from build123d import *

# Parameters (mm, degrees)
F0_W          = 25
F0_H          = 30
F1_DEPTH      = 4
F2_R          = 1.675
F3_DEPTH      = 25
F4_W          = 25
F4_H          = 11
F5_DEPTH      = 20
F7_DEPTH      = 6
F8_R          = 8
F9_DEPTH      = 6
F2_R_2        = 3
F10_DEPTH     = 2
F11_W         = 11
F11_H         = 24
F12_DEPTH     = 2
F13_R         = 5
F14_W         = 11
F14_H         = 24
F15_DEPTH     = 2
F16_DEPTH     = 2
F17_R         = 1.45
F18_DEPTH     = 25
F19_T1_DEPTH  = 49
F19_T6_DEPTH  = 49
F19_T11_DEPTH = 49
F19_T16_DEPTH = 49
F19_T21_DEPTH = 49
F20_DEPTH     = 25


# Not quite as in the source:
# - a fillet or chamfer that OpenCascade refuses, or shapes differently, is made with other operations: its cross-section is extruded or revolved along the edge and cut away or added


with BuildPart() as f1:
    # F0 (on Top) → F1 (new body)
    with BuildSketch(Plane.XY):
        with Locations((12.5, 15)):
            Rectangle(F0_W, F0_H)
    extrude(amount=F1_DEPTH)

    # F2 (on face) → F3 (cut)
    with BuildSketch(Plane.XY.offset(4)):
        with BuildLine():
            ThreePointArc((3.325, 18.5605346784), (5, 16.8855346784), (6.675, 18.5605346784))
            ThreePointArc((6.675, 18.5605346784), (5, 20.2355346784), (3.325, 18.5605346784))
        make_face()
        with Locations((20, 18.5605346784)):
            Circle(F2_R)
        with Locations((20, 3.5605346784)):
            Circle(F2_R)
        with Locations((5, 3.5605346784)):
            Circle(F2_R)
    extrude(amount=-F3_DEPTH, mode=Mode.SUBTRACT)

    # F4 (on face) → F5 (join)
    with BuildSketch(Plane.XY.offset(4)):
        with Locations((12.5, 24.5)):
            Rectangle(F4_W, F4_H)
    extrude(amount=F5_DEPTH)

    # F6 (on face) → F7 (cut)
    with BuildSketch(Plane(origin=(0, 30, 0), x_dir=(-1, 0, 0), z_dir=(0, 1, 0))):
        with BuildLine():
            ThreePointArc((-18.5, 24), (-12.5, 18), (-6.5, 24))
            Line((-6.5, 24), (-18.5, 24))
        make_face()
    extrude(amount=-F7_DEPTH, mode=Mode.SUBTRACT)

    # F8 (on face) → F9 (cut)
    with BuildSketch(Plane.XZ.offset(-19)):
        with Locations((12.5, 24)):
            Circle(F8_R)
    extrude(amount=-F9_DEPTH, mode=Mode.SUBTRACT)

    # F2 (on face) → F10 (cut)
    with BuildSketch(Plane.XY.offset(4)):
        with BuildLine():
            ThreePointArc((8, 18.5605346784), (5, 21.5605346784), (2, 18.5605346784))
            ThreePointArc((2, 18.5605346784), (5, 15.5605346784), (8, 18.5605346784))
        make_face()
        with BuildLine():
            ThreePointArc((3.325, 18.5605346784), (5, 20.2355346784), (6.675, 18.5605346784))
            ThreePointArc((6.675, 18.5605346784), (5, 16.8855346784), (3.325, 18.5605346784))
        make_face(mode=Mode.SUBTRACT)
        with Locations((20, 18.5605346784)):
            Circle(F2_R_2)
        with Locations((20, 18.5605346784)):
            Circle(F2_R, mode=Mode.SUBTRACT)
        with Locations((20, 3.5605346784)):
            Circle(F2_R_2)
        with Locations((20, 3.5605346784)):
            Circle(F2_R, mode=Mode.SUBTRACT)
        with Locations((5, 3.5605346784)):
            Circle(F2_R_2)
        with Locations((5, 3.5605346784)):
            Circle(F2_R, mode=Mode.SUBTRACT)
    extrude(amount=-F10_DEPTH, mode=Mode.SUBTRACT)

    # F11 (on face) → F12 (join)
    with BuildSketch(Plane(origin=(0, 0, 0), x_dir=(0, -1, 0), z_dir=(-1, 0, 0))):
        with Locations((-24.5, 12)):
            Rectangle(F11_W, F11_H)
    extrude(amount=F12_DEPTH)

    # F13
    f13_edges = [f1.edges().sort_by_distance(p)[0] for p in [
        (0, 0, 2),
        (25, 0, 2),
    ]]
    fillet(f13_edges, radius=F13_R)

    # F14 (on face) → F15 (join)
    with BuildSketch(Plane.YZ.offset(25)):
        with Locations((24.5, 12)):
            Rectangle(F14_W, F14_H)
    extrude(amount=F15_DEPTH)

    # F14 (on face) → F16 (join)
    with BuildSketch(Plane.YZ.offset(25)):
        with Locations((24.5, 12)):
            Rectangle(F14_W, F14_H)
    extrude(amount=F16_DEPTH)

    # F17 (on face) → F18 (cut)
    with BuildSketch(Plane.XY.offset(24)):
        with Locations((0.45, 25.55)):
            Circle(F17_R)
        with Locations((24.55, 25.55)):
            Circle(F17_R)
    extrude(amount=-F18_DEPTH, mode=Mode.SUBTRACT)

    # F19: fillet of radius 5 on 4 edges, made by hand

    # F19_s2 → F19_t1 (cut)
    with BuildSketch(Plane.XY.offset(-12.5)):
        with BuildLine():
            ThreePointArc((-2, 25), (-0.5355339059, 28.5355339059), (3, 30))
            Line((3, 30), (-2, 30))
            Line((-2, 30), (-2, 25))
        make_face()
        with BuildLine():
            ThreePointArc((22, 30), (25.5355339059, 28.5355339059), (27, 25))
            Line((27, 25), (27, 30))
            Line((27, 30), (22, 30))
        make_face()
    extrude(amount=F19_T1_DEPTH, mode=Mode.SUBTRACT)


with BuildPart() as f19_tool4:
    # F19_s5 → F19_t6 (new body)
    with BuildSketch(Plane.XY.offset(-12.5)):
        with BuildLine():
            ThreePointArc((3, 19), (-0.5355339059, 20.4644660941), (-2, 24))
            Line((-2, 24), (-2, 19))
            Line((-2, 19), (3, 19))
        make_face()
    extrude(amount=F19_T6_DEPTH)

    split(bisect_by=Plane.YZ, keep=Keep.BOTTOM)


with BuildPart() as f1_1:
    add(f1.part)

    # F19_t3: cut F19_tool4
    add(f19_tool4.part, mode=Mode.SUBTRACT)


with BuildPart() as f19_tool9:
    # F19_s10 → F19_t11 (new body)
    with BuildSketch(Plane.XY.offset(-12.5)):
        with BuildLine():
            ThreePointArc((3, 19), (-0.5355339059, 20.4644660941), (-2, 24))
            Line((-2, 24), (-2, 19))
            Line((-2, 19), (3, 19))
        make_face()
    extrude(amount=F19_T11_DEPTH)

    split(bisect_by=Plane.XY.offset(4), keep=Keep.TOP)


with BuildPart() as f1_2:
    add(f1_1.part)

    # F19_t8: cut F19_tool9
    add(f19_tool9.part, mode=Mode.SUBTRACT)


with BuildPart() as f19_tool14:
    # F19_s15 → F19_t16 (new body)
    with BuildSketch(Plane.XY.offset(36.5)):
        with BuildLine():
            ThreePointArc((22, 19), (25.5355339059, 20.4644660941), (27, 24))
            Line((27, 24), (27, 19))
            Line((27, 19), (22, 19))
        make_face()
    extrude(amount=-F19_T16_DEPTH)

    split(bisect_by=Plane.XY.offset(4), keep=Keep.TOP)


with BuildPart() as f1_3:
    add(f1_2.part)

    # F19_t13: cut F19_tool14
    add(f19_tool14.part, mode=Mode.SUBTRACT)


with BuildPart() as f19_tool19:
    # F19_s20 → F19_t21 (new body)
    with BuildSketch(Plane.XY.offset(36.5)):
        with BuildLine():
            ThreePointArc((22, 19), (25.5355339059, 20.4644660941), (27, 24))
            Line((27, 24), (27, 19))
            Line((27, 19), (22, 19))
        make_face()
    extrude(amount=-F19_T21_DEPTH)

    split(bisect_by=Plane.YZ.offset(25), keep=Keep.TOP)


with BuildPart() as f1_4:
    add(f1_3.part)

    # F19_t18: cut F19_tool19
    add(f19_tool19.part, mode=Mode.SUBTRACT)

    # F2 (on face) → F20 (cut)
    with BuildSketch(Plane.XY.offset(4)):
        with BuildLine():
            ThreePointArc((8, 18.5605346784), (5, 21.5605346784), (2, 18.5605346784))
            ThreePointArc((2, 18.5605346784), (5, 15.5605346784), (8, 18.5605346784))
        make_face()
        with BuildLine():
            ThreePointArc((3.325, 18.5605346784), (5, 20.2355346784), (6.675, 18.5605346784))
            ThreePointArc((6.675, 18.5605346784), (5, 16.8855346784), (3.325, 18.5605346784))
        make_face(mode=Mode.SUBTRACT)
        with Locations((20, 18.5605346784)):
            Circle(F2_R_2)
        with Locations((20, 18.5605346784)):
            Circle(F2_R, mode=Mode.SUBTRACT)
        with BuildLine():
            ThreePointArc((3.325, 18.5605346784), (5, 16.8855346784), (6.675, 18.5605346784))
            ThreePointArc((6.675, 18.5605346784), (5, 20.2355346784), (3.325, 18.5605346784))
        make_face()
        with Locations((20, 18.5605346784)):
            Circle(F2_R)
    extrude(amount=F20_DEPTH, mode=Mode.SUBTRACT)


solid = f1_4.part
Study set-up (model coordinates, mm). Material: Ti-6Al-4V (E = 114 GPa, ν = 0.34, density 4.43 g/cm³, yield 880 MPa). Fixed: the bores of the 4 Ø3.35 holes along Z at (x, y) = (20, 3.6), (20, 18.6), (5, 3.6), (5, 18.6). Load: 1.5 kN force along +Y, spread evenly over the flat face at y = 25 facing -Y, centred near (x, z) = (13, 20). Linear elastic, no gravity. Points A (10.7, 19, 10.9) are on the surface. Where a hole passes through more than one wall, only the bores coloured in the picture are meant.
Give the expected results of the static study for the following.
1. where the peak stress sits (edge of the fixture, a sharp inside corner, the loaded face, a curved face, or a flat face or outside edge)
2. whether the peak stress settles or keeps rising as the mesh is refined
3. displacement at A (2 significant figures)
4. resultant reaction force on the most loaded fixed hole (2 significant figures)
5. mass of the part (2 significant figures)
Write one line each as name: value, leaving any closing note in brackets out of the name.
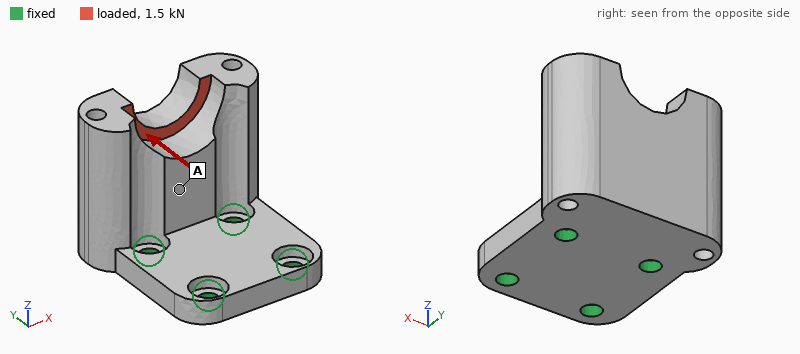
where the peak stress sits: edge of the fixture
whether the peak stress settles or keeps rising as the mesh is refined: keeps rising
displacement at A: 0.089 mm
resultant reaction force on the most loaded fixed hole: 1.3 kN
mass of the part: 31 g
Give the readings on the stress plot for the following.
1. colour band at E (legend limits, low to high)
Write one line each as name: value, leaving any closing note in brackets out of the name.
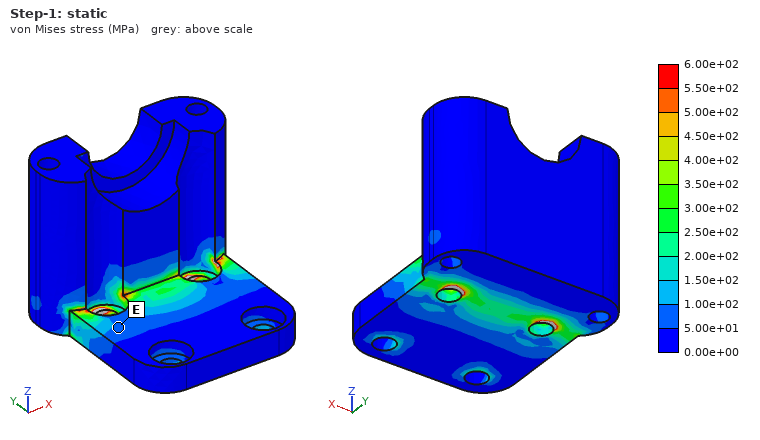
colour band at E: 5.00e+01 to 1.00e+02 MPa
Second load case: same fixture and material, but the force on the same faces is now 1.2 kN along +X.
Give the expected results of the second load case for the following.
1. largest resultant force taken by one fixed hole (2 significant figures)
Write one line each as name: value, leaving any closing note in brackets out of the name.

largest resultant force taken by one fixed hole: 1.5 kN
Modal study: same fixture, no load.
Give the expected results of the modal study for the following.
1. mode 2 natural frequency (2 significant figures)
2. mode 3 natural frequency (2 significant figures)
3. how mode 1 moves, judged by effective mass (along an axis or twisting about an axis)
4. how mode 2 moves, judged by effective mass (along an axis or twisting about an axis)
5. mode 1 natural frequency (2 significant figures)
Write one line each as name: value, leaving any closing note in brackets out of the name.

mode 2 natural frequency: 10 kHz
mode 3 natural frequency: 17 kHz
how mode 1 moves, judged by effective mass: along Y
how mode 2 moves, judged by effective mass: along X
mode 1 natural frequency: 4300 Hz
